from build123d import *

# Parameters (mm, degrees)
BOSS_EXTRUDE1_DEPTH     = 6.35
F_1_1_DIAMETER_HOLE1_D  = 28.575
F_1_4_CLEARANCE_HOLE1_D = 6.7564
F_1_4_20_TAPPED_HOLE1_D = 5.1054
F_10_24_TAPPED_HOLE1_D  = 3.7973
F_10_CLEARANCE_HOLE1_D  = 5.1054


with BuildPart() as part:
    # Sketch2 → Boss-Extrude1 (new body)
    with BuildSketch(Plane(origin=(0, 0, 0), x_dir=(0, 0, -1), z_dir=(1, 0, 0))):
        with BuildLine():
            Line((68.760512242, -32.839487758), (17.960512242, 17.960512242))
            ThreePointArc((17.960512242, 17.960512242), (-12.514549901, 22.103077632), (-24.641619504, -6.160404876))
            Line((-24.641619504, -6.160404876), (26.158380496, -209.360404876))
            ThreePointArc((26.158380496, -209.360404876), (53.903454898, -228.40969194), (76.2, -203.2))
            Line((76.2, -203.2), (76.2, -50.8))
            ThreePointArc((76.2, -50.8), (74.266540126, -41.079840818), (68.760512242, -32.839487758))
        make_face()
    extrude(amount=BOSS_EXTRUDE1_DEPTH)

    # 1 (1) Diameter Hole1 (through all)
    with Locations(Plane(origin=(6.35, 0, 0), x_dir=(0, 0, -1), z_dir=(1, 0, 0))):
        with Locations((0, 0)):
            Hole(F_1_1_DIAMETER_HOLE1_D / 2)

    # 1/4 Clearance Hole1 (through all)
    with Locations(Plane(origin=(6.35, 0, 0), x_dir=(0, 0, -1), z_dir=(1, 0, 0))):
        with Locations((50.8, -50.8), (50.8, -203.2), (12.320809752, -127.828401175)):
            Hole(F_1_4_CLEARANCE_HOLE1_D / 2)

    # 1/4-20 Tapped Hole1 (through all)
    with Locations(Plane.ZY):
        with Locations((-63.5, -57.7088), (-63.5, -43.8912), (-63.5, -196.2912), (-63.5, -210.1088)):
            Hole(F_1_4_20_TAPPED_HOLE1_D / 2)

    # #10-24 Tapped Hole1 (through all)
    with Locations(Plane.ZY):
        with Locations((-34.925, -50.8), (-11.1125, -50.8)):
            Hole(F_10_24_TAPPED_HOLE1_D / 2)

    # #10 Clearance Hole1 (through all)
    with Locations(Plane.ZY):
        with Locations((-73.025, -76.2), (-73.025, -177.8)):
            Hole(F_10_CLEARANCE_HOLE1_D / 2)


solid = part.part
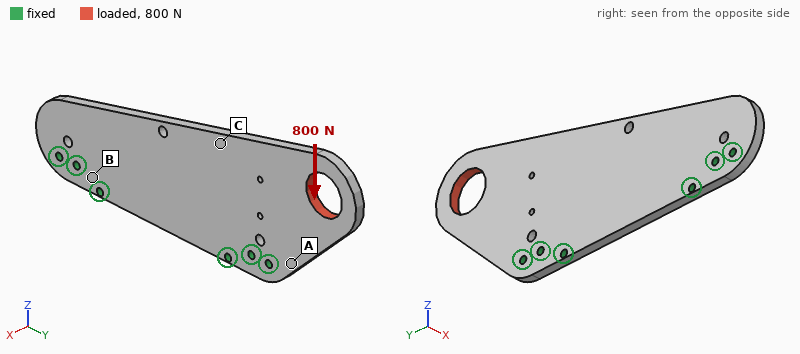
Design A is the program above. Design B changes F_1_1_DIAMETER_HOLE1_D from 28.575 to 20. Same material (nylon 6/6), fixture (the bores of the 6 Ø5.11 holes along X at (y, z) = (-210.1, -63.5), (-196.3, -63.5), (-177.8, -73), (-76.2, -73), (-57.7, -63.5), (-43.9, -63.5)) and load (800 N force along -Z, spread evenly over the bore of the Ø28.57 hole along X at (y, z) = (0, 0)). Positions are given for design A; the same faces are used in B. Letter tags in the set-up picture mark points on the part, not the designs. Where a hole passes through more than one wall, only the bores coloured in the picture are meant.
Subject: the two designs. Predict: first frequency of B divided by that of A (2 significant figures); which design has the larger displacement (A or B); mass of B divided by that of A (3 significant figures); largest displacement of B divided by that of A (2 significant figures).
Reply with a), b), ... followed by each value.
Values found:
a) 0.94
b) A
c) 1.02
d) 0.84
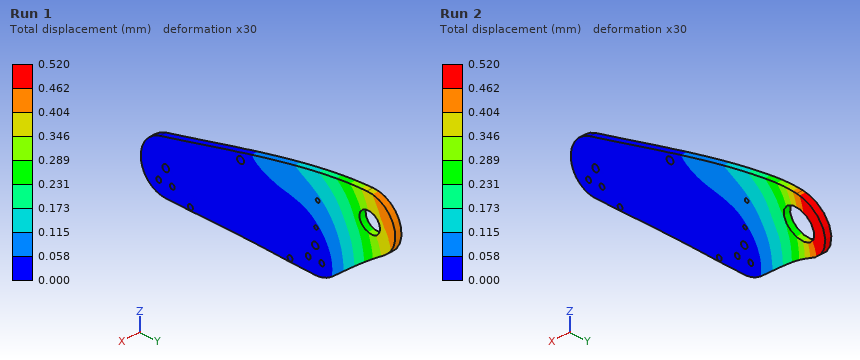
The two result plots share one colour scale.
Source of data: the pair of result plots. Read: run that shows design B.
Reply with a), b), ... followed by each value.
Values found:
a) Run 1
